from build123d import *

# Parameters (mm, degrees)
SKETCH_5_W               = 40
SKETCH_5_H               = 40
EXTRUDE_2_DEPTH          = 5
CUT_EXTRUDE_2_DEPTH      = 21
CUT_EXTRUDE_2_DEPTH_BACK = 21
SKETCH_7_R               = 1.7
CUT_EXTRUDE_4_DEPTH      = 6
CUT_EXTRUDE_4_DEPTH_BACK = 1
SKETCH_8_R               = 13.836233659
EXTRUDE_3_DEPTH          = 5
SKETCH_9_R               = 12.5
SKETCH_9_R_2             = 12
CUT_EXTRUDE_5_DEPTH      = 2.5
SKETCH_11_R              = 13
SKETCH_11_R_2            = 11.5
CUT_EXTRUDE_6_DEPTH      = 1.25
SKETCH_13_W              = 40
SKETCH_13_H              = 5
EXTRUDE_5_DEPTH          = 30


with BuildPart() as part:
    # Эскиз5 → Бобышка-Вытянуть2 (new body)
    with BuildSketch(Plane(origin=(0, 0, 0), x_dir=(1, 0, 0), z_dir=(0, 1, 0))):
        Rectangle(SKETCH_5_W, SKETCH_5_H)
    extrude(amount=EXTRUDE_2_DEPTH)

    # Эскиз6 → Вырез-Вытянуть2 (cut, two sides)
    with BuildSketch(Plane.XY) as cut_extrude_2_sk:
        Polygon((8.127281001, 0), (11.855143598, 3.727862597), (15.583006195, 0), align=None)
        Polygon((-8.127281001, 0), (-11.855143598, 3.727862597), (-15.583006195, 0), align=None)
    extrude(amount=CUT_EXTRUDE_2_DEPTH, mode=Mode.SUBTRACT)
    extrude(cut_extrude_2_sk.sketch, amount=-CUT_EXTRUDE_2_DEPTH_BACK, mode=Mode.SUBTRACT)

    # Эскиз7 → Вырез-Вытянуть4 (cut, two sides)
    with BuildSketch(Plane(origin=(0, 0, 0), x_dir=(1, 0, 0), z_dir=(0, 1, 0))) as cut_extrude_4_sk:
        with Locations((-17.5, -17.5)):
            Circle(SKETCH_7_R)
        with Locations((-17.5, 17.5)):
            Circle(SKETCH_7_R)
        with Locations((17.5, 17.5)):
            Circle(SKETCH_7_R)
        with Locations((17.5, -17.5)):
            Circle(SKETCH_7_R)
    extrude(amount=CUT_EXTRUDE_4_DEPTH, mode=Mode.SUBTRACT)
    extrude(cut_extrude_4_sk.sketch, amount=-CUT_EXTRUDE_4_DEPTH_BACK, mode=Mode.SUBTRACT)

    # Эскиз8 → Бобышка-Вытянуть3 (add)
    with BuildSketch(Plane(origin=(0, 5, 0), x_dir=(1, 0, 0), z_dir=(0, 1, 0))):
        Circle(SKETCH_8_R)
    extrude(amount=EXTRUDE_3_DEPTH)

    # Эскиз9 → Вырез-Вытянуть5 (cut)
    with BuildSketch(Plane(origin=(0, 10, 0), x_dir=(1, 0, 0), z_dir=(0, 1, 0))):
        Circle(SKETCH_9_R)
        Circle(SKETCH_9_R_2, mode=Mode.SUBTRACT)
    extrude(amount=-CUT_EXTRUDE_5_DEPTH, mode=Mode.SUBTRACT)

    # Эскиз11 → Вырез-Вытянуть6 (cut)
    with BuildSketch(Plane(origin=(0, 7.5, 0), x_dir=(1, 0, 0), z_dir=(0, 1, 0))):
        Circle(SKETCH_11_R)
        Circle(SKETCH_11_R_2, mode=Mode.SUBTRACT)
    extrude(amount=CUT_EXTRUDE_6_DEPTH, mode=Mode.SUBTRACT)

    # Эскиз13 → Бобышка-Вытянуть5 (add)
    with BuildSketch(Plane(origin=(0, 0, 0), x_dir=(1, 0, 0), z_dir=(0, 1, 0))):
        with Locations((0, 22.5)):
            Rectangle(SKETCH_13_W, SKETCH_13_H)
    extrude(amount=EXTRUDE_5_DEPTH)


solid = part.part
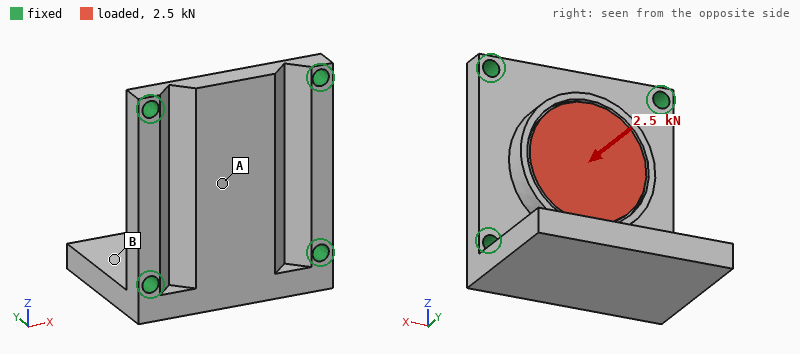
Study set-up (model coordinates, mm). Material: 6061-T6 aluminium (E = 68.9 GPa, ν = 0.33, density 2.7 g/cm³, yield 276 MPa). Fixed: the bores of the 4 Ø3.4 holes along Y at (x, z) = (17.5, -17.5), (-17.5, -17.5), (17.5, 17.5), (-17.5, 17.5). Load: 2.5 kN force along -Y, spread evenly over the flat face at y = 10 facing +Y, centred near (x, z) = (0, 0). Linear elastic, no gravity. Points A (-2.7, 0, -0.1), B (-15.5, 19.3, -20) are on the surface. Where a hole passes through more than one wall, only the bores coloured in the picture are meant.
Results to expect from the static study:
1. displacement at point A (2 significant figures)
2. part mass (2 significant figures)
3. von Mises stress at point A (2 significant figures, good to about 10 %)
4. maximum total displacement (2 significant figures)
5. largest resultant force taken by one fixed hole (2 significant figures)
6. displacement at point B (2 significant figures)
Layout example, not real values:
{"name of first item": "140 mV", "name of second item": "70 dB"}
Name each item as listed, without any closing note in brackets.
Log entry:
{"displacement at point A": "25 µm", "part mass": "42 g", "von Mises stress at point A": "19 MPa", "maximum total displacement": "27 µm", "largest resultant force taken by one fixed hole": "690 N", "displacement at point B": "14 µm"}
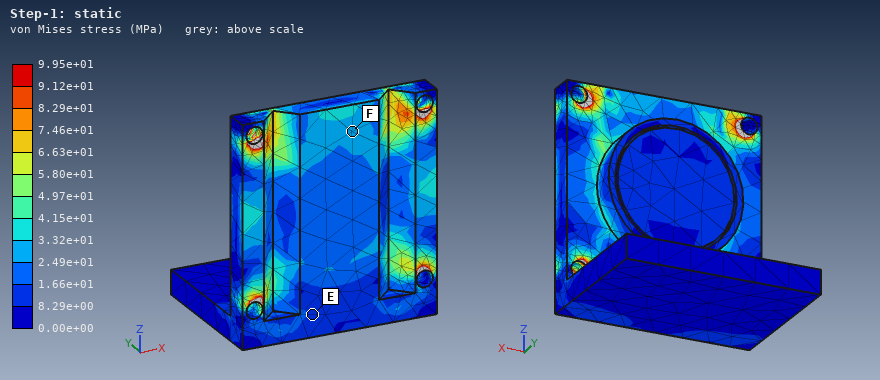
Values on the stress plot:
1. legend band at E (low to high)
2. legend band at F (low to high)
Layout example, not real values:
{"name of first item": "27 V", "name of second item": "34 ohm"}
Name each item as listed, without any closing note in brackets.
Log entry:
{"legend band at E": "8.29e+00 to 1.66e+01 MPa", "legend band at F": "2.49e+01 to 3.32e+01 MPa"}
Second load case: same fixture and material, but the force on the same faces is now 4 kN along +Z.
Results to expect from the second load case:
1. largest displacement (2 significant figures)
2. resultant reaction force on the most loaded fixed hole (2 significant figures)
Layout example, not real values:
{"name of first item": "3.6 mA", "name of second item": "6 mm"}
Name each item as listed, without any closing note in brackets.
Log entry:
{"largest displacement": "23 µm", "resultant reaction force on the most loaded fixed hole": "1.2 kN"}
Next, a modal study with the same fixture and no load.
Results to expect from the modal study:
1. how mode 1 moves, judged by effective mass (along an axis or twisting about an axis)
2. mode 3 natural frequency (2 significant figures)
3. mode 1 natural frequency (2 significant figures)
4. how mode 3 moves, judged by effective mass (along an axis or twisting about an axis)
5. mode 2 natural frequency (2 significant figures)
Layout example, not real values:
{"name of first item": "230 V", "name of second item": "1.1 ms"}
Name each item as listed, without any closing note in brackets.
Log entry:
{"how mode 1 moves, judged by effective mass": "along Z", "mode 3 natural frequency": "12 kHz", "mode 1 natural frequency": "4000 Hz", "how mode 3 moves, judged by effective mass": "along Y", "mode 2 natural frequency": "8600 Hz"}
